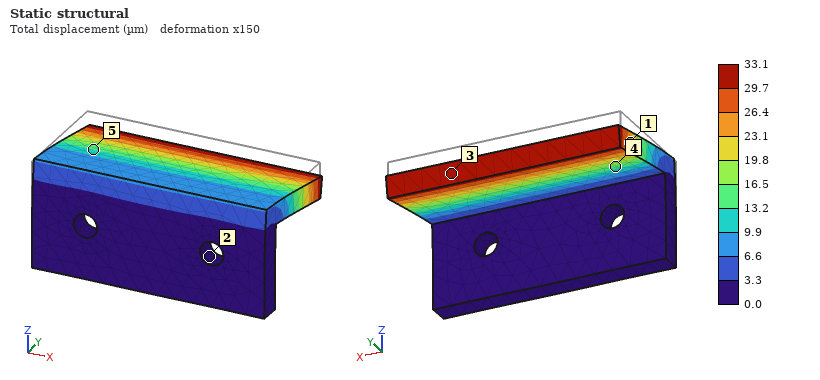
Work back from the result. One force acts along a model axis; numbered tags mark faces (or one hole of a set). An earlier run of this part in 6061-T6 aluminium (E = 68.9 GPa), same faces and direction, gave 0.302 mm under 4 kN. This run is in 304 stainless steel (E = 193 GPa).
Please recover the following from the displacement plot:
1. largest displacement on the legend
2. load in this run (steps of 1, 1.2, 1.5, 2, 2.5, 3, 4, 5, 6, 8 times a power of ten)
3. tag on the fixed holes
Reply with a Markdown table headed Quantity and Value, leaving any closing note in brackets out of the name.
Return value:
| Quantity | Value |
|---|---|
| largest displacement on the legend | 33.1 µm |
| load in this run | 1.2 kN |
| tag on the fixed holes | 2 |
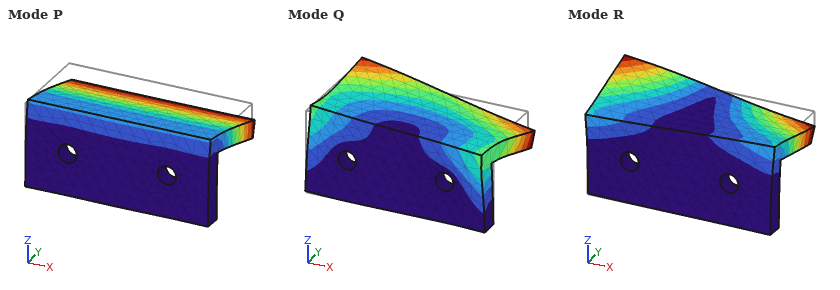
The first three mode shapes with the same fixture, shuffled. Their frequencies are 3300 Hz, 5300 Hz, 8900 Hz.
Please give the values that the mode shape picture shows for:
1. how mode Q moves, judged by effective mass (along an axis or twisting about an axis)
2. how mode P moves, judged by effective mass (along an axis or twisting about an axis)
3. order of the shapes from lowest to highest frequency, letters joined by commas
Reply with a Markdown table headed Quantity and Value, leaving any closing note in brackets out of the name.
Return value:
| Quantity | Value |
|---|---|
| how mode Q moves, judged by effective mass | along X |
| how mode P moves, judged by effective mass | along Z |
| order of the shapes from lowest to highest frequency, letters joined by commas | P, R, Q |
